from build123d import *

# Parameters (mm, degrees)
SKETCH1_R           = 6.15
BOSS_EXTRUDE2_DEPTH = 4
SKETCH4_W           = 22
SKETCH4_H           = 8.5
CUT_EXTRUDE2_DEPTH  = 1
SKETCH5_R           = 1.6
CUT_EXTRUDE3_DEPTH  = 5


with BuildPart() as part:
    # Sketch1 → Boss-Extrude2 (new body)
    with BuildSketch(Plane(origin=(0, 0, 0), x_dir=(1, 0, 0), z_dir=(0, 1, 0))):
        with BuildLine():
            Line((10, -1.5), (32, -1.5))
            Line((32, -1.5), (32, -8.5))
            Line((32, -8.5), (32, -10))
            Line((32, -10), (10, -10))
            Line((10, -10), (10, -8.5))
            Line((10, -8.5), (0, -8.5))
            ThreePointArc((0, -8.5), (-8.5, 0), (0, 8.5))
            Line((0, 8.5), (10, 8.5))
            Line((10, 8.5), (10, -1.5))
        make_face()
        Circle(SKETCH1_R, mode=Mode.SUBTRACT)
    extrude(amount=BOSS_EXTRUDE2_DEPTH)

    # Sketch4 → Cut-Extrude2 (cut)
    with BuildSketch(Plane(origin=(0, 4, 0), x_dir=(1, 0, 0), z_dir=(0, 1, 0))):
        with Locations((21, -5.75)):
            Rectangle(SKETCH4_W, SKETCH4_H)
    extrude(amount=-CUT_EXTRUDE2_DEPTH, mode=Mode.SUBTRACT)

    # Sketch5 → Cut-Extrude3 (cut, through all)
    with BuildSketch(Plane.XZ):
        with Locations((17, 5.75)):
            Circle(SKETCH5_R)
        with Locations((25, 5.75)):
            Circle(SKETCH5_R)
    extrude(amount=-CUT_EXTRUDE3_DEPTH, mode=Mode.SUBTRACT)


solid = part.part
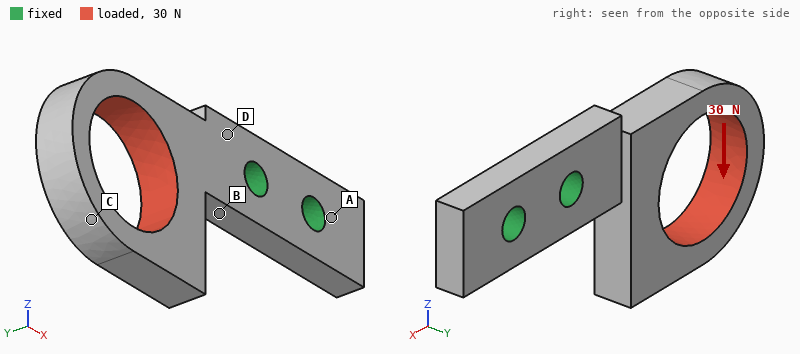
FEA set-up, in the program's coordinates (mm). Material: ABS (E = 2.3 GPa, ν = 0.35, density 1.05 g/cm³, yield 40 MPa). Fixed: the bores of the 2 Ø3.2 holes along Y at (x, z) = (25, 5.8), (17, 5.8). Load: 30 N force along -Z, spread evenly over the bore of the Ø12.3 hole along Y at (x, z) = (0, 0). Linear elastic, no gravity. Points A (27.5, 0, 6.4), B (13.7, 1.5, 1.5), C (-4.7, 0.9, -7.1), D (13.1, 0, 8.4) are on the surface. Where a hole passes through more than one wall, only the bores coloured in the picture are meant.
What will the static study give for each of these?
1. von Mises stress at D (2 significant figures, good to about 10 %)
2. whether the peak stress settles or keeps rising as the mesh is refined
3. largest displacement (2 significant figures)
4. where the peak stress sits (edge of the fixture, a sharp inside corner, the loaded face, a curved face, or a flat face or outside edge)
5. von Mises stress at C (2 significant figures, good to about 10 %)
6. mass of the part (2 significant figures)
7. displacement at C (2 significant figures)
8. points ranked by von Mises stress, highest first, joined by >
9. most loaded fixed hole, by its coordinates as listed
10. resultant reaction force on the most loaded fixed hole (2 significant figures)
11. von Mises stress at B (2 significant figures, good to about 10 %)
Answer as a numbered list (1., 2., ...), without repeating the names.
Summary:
1. 7.7 MPa
2. keeps rising
3. 0.51 mm
4. a sharp inside corner
5. 3.6 MPa
6. 1.2 g
7. 0.49 mm
8. B > D > C > A
9. (17, 5.8)
10. 53 N
11. 12 MPa
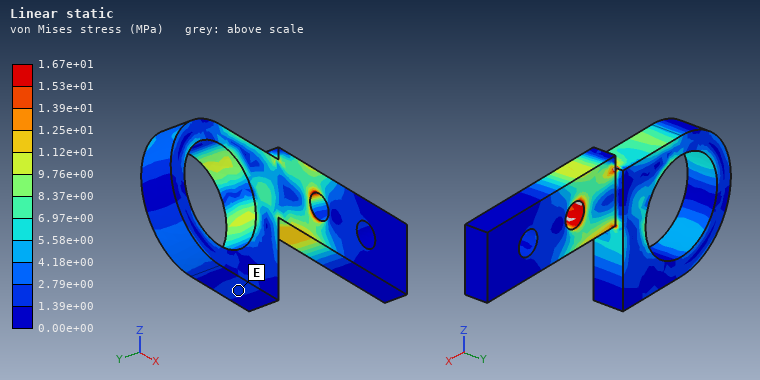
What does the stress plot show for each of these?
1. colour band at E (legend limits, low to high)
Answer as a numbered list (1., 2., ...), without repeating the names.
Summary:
1. 1.39e+00 to 2.79e+00 MPa
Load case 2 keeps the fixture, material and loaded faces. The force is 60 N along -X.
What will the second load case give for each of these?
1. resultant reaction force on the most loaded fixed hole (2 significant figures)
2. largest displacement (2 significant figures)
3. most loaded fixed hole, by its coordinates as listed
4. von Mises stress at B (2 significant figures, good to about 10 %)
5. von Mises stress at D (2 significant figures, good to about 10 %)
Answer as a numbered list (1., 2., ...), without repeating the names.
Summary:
1. 57 N
2. 0.49 mm
3. (17, 5.8)
4. 11 MPa
5. 6.4 MPa
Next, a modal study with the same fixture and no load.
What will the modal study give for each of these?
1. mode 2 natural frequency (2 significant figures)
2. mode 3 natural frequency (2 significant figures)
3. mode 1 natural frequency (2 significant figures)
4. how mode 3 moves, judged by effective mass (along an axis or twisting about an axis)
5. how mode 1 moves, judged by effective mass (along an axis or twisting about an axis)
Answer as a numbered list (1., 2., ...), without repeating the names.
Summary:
1. 1800 Hz
2. 2400 Hz
3. 1000 Hz
4. twisting about X
5. along Y
